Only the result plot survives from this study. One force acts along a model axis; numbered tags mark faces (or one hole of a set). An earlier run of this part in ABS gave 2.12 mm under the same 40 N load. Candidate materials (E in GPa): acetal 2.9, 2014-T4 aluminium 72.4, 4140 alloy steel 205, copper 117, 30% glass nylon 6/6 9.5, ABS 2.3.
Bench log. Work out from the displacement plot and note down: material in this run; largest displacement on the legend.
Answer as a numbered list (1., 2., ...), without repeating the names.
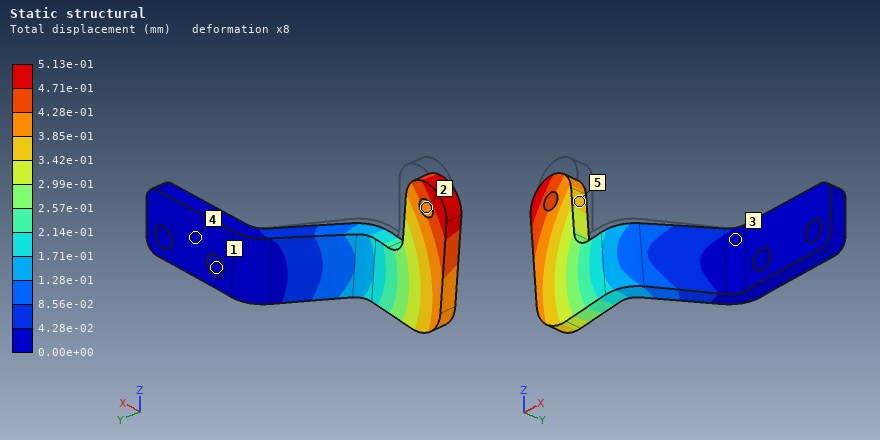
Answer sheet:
1. 30% glass nylon 6/6
2. 5.13e-01 mm
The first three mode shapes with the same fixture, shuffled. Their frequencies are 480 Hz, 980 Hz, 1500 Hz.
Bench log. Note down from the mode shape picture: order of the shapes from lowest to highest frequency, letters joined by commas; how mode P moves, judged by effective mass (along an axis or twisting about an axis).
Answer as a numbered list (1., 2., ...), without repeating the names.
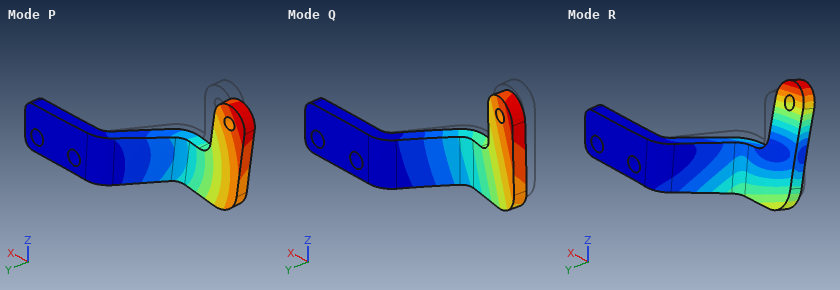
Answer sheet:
1. Q, P, R
2. along Z
